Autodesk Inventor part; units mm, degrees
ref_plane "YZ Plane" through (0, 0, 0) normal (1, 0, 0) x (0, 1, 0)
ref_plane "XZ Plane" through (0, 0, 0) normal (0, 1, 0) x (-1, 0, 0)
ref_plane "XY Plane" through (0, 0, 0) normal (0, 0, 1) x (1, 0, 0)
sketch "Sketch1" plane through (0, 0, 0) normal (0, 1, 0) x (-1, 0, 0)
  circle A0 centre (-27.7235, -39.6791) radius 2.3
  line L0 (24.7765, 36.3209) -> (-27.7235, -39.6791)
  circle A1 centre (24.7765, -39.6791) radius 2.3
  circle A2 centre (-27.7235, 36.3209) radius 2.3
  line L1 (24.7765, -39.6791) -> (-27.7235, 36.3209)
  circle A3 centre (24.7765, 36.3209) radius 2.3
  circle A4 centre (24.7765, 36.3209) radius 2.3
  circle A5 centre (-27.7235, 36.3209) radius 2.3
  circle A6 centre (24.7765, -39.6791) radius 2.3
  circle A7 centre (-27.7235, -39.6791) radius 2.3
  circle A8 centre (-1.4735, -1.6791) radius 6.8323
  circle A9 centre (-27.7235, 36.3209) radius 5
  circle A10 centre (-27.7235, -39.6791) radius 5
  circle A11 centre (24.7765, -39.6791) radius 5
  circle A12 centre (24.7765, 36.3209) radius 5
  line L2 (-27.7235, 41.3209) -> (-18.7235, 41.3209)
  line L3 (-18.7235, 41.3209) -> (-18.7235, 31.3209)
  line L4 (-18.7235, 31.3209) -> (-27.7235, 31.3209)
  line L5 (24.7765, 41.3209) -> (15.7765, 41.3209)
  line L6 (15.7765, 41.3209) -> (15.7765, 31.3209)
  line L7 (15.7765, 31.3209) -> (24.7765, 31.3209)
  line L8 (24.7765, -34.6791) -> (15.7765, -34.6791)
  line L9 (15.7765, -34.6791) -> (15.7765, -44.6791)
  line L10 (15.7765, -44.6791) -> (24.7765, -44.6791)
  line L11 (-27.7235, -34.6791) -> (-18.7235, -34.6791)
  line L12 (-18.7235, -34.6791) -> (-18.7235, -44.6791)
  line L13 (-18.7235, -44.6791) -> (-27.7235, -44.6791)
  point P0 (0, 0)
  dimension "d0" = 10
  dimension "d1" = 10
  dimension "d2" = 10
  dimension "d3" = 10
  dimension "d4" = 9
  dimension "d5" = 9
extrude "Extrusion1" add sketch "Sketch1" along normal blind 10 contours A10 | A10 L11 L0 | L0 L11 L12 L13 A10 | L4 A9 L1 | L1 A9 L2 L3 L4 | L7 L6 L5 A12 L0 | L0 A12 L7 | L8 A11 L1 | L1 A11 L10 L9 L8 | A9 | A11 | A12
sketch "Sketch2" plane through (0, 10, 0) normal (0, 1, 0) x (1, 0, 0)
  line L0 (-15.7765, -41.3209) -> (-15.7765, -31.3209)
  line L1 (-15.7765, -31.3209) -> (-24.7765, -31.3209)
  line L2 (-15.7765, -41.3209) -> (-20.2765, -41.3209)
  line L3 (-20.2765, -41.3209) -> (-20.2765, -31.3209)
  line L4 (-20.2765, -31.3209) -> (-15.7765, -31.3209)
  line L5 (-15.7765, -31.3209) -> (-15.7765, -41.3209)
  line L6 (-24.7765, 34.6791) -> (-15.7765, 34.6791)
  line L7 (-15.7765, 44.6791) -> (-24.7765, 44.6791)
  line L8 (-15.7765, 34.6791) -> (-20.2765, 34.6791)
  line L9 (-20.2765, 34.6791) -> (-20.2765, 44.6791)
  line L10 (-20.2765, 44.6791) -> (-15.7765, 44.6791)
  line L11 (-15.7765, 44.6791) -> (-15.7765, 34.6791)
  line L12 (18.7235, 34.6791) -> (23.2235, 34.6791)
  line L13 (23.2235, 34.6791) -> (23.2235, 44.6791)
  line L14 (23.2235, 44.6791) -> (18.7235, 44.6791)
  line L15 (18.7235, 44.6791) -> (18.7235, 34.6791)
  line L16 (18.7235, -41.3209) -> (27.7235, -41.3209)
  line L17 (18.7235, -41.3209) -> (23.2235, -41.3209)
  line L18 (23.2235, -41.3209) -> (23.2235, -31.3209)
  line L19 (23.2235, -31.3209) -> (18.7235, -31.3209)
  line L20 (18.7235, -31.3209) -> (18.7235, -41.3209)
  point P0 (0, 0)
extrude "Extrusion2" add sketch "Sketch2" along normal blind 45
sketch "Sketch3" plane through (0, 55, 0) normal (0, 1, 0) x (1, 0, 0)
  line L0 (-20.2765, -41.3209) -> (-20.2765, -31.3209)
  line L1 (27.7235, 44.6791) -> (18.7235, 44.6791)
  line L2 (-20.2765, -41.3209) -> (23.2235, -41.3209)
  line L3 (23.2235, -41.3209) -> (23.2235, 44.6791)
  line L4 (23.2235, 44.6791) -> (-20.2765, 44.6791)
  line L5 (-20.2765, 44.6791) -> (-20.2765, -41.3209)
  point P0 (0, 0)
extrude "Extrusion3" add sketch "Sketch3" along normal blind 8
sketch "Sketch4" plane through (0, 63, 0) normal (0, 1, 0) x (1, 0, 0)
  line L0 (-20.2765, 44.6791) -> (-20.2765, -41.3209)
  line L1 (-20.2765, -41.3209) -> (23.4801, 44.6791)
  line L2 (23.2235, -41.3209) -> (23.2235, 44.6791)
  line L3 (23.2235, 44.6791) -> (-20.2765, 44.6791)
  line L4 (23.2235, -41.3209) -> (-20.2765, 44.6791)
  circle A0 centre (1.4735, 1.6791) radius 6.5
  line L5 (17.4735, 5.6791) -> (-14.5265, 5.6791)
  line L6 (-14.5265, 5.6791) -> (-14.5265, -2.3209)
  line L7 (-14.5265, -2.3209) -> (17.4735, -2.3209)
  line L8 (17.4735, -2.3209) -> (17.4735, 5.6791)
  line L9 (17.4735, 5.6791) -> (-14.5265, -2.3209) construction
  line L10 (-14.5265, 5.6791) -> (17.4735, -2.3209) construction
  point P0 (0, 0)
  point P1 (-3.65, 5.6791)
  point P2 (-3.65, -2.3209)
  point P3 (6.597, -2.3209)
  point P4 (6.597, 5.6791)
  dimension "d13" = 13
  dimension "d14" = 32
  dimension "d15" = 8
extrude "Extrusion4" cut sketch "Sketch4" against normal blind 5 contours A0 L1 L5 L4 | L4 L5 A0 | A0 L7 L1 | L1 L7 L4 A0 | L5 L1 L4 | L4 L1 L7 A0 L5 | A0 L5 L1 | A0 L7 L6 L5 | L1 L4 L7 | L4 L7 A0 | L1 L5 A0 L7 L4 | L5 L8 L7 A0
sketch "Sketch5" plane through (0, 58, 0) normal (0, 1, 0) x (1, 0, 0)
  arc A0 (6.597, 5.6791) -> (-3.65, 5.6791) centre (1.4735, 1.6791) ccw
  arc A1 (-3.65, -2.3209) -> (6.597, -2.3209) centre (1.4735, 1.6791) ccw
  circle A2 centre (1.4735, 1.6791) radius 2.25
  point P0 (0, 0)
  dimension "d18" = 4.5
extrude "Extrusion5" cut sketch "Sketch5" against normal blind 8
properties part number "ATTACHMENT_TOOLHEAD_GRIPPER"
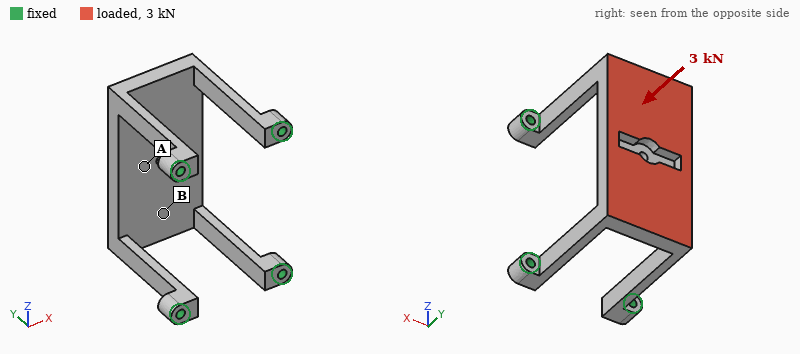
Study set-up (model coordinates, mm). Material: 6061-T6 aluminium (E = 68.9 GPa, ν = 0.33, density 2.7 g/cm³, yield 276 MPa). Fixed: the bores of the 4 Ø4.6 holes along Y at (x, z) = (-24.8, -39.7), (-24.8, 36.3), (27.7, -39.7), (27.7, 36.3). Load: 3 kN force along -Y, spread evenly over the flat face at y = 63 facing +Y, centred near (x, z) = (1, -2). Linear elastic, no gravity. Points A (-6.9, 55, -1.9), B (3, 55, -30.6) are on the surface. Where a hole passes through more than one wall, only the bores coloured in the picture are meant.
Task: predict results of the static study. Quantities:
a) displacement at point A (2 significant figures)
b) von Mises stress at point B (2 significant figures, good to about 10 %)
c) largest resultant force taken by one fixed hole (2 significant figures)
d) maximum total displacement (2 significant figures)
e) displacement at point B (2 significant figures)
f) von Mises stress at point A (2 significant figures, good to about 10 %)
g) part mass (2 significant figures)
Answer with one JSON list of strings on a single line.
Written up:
["0.11 mm", "11 MPa", "760 N", "0.11 mm", "0.049 mm", "42 MPa", "110 g"]
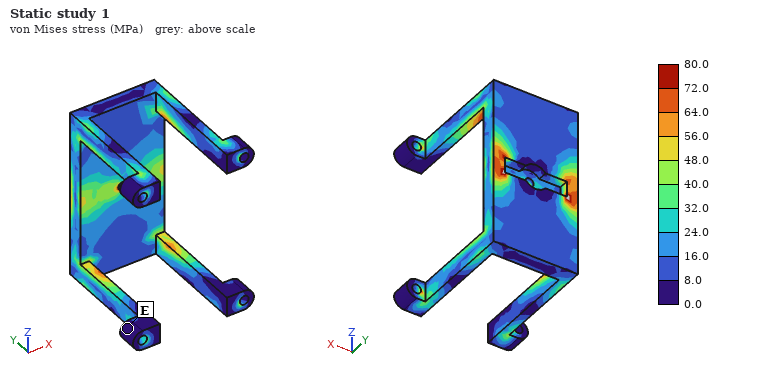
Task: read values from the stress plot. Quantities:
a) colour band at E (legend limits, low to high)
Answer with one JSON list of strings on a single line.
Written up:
["0.0 to 8.0 MPa"]
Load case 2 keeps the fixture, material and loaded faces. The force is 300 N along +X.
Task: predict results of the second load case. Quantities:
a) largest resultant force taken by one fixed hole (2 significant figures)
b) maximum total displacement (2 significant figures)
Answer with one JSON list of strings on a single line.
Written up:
["140 N", "0.15 mm"]
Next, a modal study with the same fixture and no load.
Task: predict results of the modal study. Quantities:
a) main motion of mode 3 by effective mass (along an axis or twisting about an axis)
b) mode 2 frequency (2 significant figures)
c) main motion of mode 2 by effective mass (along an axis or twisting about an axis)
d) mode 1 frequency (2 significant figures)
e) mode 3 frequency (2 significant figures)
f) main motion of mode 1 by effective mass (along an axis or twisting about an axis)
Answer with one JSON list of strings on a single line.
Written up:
["twisting about Y", "1300 Hz", "along Z", "780 Hz", "1400 Hz", "along X"]
